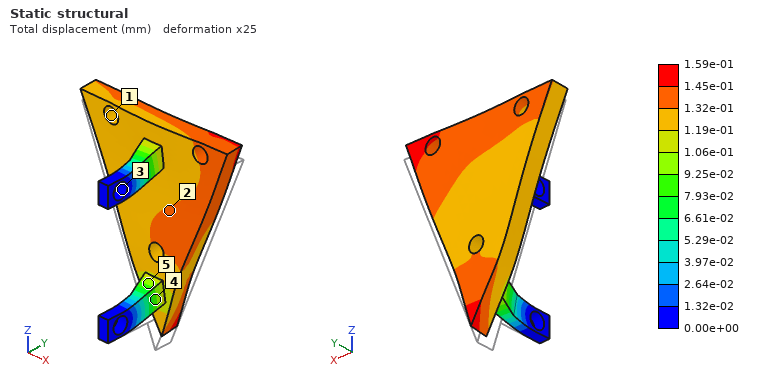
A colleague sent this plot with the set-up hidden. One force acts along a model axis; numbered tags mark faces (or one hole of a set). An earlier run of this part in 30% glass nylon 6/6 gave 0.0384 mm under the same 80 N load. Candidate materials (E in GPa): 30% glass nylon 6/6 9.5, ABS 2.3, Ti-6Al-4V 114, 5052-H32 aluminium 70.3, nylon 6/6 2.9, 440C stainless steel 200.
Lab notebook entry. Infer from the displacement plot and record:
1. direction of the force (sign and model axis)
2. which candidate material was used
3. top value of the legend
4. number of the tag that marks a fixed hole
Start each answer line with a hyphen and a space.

- +Z
- ABS
- 1.59e-01 mm
- 3
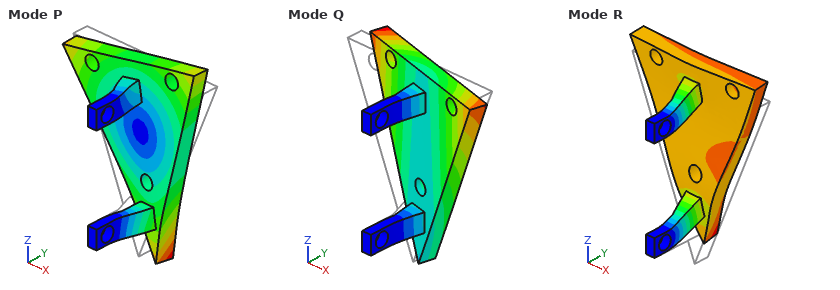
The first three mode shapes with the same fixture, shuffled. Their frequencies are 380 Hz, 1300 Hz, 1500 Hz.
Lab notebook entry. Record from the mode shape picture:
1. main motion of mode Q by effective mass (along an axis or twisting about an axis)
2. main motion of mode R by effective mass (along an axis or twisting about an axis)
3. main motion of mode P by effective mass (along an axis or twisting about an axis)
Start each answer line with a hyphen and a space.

- along X
- along Z
- twisting about Y
